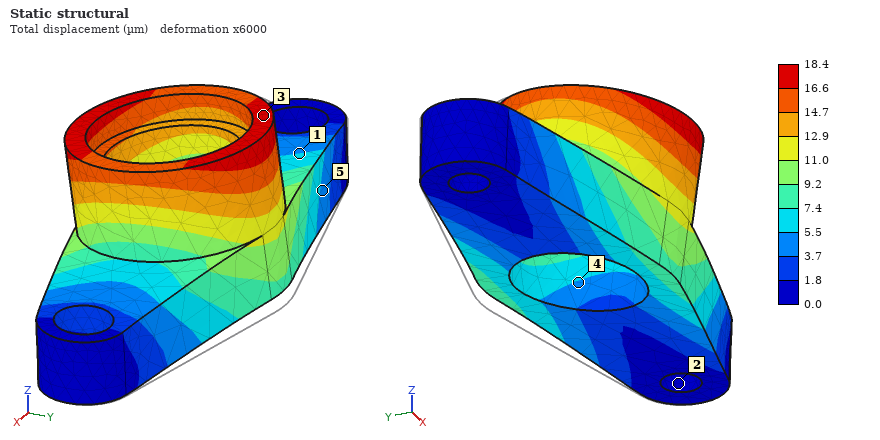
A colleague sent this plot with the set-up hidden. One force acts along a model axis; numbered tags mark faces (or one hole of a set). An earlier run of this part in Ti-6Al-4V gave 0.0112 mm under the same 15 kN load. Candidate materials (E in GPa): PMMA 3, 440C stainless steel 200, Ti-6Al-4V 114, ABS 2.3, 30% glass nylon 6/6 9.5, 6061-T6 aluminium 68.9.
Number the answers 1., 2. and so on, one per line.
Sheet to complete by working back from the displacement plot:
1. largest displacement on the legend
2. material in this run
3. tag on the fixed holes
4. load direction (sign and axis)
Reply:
1. 18.4 µm
2. 6061-T6 aluminium
3. 2
4. -Y
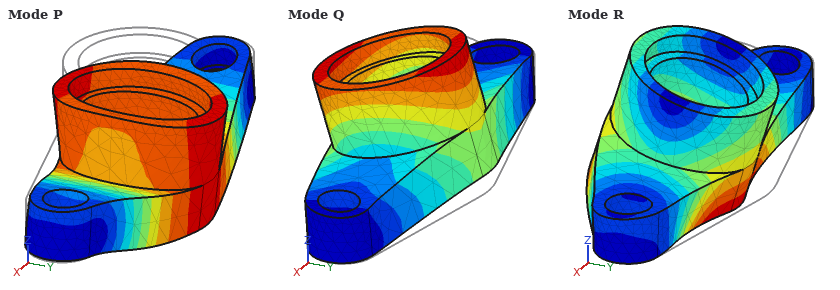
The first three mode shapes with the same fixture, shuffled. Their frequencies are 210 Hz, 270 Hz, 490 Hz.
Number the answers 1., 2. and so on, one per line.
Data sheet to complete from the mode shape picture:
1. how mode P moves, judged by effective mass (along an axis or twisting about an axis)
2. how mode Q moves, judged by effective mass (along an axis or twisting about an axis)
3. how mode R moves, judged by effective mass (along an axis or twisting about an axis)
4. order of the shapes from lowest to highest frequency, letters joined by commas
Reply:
1. along Z
2. along Y
3. along Y
4. Q, P, R
